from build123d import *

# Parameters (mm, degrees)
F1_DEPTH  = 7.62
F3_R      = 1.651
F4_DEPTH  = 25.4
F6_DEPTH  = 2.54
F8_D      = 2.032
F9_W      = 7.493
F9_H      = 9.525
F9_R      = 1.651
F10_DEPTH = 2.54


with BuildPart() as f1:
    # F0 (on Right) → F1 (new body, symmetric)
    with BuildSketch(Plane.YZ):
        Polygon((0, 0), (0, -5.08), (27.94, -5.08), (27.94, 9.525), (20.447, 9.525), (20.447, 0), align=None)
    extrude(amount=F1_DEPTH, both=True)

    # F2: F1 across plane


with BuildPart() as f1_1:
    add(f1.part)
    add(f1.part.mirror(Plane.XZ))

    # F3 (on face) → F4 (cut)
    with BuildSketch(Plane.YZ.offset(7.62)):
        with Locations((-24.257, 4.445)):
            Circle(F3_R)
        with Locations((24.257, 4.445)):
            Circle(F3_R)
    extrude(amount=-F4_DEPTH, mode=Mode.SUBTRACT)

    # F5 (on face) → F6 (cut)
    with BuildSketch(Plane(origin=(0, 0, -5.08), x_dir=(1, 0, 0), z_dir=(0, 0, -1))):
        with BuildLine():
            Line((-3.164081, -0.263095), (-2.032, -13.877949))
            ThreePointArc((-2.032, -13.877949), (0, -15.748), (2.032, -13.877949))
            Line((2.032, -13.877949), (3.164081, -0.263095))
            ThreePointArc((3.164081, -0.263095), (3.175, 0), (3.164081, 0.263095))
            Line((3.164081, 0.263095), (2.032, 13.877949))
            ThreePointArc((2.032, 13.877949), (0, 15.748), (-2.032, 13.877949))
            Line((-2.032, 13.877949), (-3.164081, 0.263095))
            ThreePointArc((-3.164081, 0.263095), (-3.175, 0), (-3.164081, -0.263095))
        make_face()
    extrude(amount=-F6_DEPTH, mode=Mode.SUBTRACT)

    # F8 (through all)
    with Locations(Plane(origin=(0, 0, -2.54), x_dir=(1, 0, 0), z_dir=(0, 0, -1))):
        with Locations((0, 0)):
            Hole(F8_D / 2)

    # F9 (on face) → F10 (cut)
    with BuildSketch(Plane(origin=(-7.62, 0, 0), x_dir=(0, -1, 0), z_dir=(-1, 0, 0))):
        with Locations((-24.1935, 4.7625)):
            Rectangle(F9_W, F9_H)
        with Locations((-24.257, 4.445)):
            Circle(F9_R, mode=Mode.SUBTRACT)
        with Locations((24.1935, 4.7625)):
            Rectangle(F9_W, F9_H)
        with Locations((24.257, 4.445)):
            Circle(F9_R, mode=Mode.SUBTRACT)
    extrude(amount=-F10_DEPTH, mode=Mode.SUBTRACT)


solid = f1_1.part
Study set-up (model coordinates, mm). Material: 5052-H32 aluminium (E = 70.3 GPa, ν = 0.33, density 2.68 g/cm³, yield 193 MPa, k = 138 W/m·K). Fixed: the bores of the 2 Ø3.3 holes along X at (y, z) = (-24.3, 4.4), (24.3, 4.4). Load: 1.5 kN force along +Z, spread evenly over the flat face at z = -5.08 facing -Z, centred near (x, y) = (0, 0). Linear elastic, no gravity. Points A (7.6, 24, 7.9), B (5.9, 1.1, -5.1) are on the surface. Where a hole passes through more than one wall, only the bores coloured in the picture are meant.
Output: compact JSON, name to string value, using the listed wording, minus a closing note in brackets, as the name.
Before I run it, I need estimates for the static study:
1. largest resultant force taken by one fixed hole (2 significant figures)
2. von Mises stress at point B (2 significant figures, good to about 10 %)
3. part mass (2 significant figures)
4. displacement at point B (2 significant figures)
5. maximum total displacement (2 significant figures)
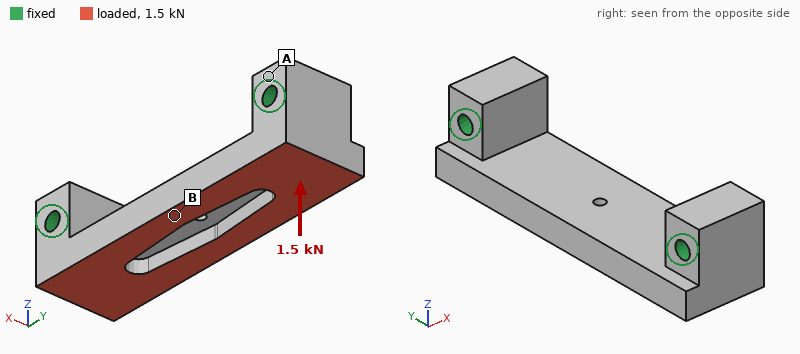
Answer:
{"largest resultant force taken by one fixed hole": "860 N", "von Mises stress at point B": "50 MPa", "part mass": "15 g", "displacement at point B": "33 µm", "maximum total displacement": "36 µm"}
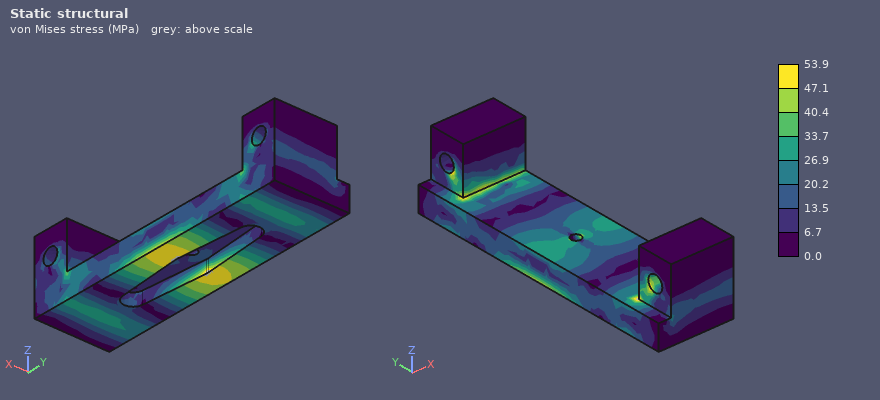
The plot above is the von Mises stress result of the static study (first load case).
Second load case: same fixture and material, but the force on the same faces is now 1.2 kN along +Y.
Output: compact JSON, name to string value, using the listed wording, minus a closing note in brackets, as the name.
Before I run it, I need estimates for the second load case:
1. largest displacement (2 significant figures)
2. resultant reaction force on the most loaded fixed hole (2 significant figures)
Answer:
{"largest displacement": "6.2 µm", "resultant reaction force on the most loaded fixed hole": "610 N"}
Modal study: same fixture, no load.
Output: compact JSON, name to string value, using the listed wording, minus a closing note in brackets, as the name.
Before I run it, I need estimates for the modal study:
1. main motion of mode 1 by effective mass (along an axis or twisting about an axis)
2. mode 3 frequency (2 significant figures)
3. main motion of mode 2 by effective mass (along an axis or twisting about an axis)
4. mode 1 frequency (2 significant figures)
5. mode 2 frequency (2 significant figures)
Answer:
{"main motion of mode 1 by effective mass": "along Z", "mode 3 frequency": "19 kHz", "main motion of mode 2 by effective mass": "along X", "mode 1 frequency": "11 kHz", "mode 2 frequency": "18 kHz"}
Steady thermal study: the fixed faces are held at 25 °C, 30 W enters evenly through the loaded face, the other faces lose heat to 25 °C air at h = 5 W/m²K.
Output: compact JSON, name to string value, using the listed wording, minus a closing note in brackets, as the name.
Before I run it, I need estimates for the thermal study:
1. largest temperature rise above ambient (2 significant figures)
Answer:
{"largest temperature rise above ambient": "18 K"}
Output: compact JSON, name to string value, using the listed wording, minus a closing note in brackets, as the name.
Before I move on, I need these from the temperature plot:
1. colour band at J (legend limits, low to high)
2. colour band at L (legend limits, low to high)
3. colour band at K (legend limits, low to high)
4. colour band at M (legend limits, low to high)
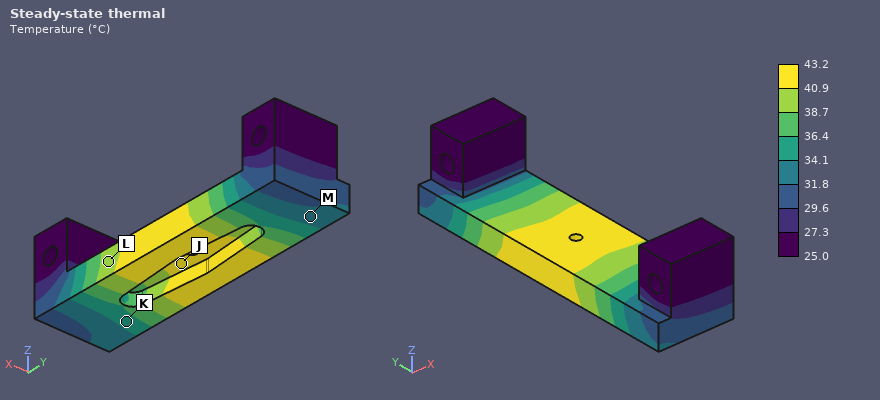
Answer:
{"colour band at J": "40.9 to 43.2 °C", "colour band at L": "38.7 to 40.9 °C", "colour band at K": "34.1 to 36.4 °C", "colour band at M": "31.8 to 34.1 °C"}
